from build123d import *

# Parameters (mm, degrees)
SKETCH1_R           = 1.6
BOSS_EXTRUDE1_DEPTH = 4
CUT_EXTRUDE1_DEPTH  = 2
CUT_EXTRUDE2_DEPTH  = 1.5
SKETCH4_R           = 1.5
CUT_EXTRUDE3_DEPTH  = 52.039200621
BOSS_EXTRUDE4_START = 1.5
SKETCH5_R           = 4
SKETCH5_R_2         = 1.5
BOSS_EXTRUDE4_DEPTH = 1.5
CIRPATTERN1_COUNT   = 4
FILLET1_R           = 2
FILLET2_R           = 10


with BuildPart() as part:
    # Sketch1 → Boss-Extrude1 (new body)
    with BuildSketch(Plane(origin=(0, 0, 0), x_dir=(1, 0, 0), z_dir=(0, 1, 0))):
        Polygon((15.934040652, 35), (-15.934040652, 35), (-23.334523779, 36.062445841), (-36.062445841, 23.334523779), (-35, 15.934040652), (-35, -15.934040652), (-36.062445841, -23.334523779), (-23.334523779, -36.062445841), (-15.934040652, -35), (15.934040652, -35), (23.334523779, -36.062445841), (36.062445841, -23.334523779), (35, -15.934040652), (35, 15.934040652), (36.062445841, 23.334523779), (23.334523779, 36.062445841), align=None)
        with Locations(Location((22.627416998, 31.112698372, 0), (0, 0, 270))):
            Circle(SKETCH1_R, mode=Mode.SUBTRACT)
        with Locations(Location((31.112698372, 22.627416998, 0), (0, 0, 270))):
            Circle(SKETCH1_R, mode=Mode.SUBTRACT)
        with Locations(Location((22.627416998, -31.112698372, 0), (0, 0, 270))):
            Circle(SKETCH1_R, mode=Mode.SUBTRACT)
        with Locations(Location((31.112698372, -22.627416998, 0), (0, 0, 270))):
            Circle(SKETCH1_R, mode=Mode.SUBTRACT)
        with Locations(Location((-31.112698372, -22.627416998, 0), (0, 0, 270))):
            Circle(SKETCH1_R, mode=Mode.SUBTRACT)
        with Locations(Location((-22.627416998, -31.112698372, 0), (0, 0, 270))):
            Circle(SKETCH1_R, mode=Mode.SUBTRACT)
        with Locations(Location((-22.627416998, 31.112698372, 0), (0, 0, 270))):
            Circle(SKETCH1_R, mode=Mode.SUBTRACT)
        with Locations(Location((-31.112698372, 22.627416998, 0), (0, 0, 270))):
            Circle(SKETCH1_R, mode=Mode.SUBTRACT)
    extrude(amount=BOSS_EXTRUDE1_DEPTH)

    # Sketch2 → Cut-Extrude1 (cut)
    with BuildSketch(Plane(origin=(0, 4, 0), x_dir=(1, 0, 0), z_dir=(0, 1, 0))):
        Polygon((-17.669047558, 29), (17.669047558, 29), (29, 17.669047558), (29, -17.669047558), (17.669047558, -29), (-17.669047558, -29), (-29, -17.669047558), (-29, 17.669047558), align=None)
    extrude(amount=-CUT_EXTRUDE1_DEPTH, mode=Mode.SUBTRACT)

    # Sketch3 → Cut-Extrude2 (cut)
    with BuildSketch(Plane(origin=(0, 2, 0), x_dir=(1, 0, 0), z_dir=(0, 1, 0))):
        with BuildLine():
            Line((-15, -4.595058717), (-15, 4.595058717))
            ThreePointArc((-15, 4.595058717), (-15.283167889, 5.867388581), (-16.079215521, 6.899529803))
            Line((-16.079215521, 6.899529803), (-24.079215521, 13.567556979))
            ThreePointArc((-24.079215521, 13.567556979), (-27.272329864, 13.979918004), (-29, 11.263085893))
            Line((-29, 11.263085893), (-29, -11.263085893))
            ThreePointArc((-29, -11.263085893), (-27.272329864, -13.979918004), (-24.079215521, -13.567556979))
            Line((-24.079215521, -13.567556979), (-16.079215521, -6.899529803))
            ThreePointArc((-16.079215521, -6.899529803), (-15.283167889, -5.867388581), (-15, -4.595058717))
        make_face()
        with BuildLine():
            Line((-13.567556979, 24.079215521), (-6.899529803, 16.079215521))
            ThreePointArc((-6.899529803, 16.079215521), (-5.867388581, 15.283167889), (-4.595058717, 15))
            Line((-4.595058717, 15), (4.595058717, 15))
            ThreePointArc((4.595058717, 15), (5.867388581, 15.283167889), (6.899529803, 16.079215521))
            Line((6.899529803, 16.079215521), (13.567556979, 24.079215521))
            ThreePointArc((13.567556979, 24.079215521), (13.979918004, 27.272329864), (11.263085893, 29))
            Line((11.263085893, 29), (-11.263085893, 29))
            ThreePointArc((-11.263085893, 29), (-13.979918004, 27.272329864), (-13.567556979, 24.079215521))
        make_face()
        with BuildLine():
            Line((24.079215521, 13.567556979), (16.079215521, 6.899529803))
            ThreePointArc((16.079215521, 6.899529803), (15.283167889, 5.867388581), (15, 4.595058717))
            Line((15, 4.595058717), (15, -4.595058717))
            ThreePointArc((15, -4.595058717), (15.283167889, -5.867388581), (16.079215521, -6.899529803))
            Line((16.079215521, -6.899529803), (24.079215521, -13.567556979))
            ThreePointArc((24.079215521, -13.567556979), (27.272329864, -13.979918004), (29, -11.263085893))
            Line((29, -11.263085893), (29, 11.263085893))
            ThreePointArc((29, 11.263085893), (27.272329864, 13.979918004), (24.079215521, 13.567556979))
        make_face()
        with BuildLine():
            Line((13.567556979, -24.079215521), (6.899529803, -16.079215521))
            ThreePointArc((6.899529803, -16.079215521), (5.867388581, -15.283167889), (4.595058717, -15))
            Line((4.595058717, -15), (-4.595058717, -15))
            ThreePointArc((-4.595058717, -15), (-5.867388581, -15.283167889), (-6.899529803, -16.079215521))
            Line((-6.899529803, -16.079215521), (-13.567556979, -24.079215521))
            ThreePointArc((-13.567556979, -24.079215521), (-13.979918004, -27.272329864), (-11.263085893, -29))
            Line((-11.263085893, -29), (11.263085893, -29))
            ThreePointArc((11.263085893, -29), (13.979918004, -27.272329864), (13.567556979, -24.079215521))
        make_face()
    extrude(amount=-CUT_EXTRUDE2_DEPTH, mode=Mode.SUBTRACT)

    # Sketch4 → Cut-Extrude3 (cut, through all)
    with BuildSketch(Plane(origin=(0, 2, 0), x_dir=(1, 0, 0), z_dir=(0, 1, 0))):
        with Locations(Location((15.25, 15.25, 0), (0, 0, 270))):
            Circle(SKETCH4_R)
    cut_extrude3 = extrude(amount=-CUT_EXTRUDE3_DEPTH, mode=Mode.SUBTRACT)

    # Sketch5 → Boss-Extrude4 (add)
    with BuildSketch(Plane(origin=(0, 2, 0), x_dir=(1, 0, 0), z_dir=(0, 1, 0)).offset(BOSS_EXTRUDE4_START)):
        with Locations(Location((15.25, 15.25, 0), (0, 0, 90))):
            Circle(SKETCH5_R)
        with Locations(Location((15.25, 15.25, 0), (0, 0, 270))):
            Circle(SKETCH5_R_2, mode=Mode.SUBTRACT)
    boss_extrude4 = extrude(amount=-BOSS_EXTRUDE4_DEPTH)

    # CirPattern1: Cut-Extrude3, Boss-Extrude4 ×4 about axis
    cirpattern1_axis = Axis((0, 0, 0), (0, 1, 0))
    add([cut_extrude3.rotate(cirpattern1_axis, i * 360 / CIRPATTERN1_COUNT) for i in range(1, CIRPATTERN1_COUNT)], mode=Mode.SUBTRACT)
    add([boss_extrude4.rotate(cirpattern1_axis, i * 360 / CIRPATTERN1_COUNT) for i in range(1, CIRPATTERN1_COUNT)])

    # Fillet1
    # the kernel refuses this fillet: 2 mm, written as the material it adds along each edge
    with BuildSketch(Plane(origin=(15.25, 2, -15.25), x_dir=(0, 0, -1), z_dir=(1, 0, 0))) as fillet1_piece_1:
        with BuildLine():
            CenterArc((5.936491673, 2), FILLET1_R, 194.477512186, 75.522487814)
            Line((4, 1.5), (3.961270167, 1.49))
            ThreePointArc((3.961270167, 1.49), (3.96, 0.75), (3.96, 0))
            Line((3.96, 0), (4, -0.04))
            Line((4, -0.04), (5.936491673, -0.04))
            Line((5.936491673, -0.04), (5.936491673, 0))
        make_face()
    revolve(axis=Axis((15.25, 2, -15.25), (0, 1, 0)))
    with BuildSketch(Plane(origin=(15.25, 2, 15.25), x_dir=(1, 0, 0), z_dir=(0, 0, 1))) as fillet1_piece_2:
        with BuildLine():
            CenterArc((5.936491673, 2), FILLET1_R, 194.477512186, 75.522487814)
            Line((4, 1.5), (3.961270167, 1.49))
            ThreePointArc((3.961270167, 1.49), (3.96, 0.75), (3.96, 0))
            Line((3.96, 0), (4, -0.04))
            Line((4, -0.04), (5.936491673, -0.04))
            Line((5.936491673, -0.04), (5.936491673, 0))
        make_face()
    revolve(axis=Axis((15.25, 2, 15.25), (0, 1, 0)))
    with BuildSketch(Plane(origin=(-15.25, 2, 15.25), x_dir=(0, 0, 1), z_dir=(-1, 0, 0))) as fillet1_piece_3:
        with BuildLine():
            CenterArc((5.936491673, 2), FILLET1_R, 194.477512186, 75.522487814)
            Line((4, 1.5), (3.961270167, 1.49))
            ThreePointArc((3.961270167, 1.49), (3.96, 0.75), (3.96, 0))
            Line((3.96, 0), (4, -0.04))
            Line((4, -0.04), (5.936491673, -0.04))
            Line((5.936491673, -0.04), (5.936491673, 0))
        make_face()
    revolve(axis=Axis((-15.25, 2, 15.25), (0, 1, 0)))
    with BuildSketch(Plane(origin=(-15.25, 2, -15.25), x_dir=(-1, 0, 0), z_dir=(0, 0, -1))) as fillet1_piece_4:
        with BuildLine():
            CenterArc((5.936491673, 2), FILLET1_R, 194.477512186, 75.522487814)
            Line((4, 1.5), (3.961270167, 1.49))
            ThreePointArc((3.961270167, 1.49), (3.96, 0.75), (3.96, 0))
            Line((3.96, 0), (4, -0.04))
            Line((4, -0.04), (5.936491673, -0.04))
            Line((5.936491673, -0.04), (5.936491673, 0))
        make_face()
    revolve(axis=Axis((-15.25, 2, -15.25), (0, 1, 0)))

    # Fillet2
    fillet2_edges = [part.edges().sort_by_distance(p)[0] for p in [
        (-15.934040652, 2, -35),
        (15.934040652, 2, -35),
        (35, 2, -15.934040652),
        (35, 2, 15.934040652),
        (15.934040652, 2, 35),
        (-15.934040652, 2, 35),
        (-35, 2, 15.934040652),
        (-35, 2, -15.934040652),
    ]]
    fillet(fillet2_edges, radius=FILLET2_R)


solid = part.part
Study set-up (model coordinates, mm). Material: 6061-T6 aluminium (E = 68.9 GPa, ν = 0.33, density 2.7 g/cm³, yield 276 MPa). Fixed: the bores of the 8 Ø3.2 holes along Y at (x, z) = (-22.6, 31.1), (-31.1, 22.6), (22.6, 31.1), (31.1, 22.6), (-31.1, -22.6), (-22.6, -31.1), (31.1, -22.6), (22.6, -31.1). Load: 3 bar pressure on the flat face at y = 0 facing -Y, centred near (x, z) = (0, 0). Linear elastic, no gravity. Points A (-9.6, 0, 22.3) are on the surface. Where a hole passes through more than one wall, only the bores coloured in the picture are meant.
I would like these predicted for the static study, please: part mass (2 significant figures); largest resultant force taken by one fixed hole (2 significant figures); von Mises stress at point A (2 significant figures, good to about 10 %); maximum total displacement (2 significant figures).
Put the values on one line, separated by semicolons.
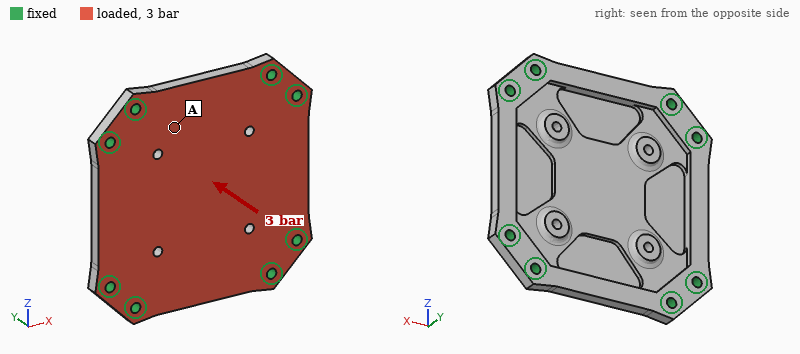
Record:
29 g; 210 N; 36 MPa; 0.22 mm
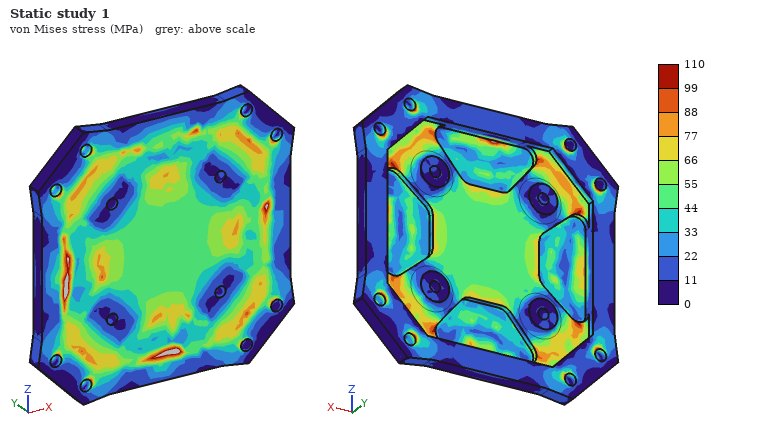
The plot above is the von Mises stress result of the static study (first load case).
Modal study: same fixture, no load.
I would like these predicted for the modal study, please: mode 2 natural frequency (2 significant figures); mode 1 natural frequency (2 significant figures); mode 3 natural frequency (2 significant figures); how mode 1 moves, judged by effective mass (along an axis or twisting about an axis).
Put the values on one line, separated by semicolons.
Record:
7200 Hz; 3300 Hz; 7200 Hz; along Y
